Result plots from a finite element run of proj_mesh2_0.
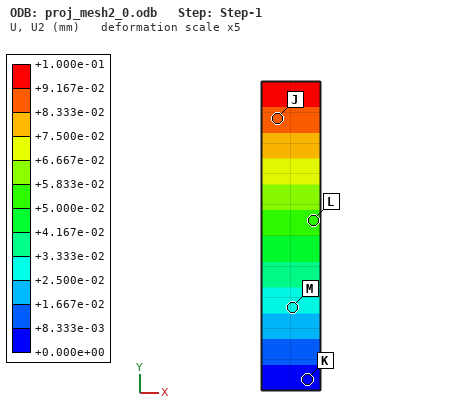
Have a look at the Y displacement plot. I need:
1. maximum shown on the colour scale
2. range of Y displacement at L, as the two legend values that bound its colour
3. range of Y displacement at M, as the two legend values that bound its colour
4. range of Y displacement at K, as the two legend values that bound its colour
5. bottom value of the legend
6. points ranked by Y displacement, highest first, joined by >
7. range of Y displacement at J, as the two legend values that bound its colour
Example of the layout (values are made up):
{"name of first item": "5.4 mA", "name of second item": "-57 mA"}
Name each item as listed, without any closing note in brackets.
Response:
{"maximum shown on the colour scale": "+1.000e-01 mm", "range of Y displacement at L, as the two legend values that bound its colour": "+5.000e-02 to +5.833e-02 mm", "range of Y displacement at M, as the two legend values that bound its colour": "+2.500e-02 to +3.333e-02 mm", "range of Y displacement at K, as the two legend values that bound its colour": "+0.000e+00 to +8.333e-03 mm", "bottom value of the legend": "+0.000e+00 mm", "points ranked by Y displacement, highest first, joined by >": "J > L > M > K", "range of Y displacement at J, as the two legend values that bound its colour": "+8.333e-02 to +9.167e-02 mm"}
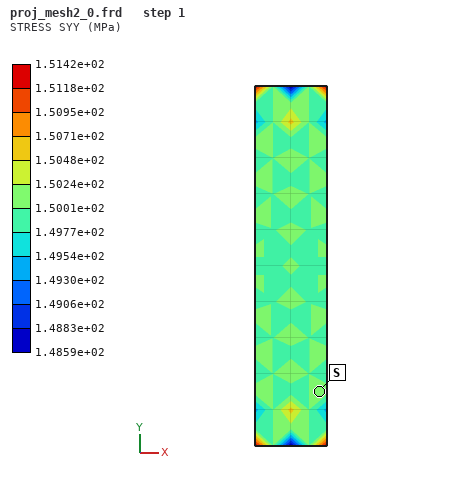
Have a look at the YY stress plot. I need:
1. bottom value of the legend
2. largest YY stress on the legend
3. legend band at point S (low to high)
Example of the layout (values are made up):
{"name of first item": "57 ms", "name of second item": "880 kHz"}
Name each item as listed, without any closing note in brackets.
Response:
{"bottom value of the legend": "1.4859e+02 MPa", "largest YY stress on the legend": "1.5142e+02 MPa", "legend band at point S": "1.5001e+02 to 1.5024e+02 MPa"}
